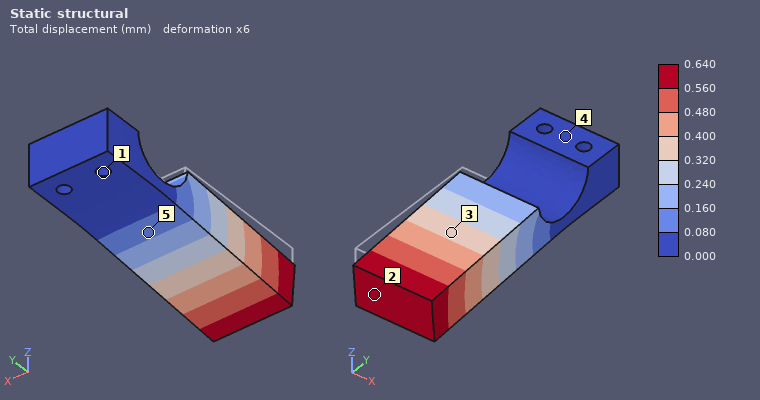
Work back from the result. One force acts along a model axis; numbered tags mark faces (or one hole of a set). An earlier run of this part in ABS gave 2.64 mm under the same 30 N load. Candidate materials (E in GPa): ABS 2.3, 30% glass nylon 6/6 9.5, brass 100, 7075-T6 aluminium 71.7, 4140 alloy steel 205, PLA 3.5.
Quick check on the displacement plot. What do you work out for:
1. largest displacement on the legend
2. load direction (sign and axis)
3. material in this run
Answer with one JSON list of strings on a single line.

["0.640 mm", "-Z", "30% glass nylon 6/6"]
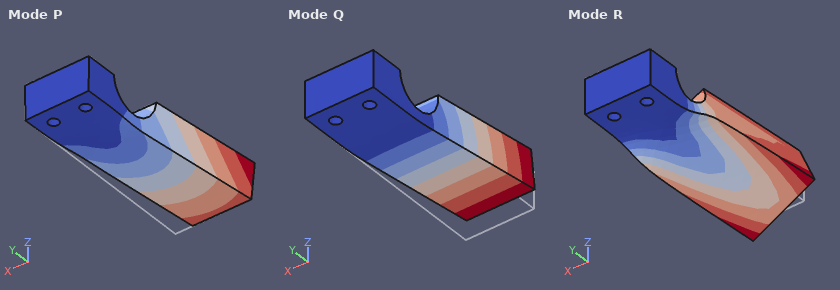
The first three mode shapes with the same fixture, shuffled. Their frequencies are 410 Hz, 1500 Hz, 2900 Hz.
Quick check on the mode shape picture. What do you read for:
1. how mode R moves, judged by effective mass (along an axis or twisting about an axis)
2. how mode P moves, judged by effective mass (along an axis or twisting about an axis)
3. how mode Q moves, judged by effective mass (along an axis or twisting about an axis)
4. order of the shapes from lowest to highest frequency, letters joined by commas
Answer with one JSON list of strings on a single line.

["twisting about Y", "along X", "along Z", "Q, P, R"]
